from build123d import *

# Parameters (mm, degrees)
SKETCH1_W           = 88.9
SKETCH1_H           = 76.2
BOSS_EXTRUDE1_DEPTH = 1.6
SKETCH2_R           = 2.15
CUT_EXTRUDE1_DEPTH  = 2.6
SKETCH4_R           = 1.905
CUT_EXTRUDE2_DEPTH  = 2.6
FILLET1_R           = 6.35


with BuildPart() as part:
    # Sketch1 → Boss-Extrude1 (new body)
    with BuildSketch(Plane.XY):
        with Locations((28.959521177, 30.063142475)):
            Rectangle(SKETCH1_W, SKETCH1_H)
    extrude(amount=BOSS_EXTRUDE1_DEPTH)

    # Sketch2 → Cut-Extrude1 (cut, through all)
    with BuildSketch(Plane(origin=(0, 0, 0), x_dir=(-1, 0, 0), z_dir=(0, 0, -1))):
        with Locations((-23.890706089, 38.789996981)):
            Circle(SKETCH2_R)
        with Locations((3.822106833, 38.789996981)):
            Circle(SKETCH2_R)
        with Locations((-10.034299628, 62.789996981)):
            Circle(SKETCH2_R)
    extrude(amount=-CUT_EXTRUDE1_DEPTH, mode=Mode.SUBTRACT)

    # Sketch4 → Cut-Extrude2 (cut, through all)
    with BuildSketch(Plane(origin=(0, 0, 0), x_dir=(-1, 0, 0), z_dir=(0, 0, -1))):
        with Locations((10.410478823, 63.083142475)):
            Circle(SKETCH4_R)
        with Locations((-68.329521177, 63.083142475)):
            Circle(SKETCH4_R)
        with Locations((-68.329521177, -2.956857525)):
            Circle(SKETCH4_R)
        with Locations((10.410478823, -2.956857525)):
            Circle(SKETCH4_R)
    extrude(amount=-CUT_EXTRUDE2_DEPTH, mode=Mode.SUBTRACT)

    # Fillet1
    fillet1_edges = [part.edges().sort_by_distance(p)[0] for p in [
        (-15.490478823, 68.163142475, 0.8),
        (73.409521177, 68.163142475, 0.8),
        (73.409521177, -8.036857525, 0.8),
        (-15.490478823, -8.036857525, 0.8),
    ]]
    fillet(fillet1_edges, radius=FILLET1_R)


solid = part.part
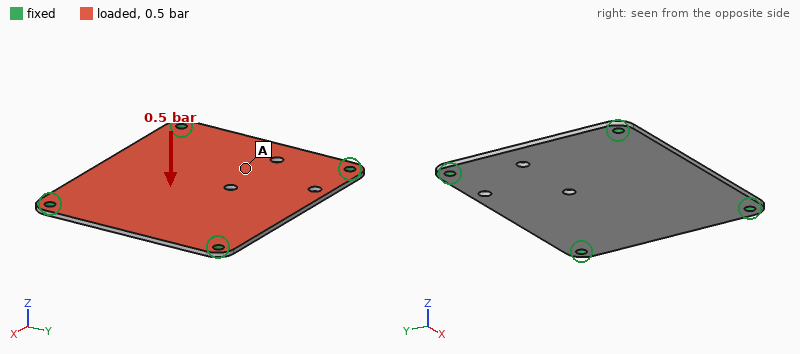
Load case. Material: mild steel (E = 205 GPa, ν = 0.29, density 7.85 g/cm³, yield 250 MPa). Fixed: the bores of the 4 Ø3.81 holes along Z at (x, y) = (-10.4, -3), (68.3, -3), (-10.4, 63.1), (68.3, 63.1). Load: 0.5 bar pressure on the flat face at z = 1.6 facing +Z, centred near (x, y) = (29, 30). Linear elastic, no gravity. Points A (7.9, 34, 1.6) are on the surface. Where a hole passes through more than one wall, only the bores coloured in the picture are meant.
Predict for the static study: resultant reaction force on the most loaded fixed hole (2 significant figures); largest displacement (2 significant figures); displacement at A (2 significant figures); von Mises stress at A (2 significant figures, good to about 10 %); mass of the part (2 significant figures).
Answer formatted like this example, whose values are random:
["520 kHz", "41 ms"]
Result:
["84 N", "0.14 mm", "0.11 mm", "26 MPa", "84 g"]
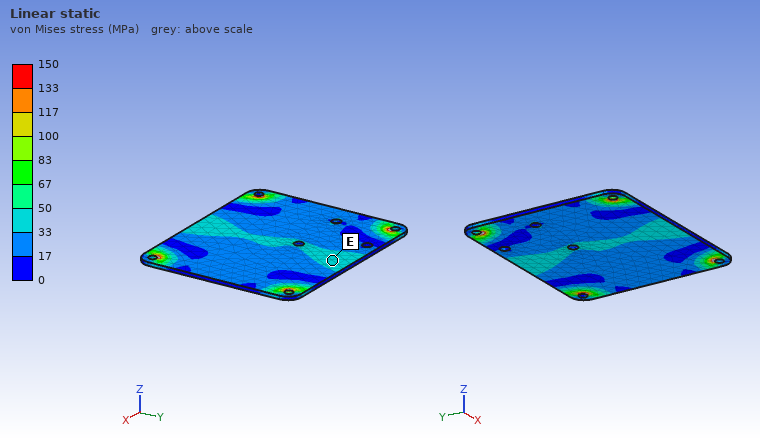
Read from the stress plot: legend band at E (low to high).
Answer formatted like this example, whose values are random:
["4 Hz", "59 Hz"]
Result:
["33 to 50 MPa"]
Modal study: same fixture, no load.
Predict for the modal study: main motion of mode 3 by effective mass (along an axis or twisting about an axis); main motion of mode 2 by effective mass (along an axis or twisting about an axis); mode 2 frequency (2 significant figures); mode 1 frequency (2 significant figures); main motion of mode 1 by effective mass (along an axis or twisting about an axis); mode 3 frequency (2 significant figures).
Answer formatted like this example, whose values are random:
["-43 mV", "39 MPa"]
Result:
["twisting about Y", "twisting about X", "1700 Hz", "1000 Hz", "along Z", "2000 Hz"]
